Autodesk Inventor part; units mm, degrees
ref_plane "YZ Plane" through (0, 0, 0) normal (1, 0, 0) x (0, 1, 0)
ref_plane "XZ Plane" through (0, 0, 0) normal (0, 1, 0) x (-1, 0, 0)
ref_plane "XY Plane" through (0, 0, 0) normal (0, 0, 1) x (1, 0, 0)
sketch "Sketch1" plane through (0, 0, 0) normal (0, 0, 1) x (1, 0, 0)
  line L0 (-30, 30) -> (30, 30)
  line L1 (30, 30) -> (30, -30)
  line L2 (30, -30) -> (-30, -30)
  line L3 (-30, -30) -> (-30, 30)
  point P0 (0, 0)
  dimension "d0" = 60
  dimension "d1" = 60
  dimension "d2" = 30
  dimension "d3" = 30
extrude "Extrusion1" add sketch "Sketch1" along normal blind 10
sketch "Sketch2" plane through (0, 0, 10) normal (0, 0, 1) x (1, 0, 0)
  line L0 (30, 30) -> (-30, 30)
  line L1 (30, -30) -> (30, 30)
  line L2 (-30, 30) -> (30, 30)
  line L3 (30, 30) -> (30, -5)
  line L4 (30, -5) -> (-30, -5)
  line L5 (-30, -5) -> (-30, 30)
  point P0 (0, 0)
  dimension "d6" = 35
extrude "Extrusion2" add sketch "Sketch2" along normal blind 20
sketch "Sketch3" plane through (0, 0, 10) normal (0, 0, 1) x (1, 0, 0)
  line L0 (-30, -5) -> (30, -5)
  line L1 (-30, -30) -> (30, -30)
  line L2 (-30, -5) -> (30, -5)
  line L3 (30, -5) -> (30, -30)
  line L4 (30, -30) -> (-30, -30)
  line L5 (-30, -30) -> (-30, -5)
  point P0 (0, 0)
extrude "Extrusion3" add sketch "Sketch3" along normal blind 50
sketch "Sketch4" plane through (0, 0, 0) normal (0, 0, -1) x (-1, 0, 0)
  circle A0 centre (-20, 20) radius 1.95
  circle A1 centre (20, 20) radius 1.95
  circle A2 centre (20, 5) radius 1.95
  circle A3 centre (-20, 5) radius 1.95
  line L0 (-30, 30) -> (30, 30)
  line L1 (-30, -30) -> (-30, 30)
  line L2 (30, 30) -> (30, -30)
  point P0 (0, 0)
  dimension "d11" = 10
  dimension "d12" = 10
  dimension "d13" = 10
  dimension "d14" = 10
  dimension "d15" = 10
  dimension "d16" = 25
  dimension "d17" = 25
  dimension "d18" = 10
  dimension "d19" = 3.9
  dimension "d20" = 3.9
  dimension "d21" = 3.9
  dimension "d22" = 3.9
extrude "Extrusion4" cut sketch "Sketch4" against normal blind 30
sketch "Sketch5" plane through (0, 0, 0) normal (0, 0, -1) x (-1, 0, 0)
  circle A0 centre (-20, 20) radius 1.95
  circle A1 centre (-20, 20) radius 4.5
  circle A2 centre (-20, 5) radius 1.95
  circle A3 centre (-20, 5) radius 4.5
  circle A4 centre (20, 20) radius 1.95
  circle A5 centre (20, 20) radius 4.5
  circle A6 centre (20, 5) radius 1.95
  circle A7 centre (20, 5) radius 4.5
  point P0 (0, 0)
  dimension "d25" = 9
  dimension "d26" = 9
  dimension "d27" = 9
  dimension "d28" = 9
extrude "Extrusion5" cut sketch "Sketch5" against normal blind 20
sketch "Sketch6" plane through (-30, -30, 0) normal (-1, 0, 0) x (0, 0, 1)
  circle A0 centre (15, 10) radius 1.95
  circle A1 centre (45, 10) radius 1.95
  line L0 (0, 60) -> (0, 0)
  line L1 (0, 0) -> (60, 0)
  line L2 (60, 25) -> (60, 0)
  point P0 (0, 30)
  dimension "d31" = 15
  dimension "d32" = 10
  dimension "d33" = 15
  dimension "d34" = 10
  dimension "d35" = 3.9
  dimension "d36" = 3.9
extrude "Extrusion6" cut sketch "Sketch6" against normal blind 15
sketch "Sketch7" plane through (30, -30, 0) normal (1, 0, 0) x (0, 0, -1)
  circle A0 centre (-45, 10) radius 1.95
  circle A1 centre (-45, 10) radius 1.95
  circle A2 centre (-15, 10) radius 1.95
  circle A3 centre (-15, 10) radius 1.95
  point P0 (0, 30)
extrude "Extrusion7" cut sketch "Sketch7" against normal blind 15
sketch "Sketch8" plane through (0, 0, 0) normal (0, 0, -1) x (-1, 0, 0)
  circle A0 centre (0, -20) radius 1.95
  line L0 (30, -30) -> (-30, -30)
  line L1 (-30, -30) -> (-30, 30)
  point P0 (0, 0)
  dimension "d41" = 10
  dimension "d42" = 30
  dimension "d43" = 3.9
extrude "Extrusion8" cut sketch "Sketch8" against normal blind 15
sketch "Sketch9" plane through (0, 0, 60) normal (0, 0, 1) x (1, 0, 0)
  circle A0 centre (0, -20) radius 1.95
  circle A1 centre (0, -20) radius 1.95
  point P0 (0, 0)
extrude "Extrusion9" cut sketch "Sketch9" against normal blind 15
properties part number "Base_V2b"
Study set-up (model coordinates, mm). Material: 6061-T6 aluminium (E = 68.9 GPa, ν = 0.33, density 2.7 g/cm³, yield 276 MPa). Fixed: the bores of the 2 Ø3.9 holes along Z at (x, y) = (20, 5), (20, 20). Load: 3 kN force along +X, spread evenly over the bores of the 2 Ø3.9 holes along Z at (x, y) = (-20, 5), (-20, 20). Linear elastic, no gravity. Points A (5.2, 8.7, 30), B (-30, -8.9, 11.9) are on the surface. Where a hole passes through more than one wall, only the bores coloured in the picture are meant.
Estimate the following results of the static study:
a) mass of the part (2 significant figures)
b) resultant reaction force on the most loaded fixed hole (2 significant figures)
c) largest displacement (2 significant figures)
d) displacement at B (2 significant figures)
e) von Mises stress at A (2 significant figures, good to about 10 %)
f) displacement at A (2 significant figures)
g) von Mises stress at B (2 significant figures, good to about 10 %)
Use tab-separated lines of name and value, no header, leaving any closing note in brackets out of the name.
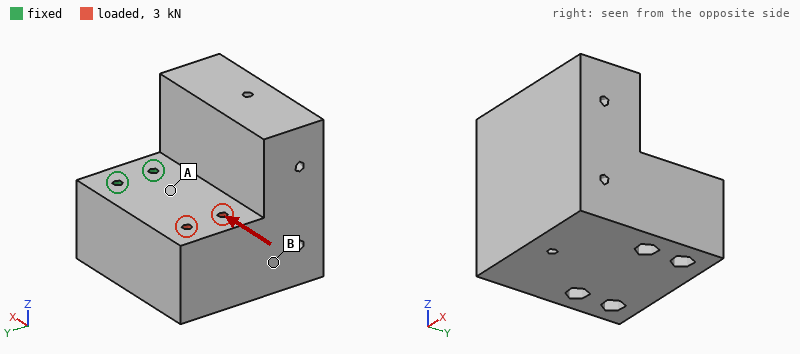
mass of the part	400 g
resultant reaction force on the most loaded fixed hole	1.5 kN
largest displacement	7.0 µm
displacement at B	3.8 µm
von Mises stress at A	7.9 MPa
displacement at A	2.0 µm
von Mises stress at B	2.1 MPa
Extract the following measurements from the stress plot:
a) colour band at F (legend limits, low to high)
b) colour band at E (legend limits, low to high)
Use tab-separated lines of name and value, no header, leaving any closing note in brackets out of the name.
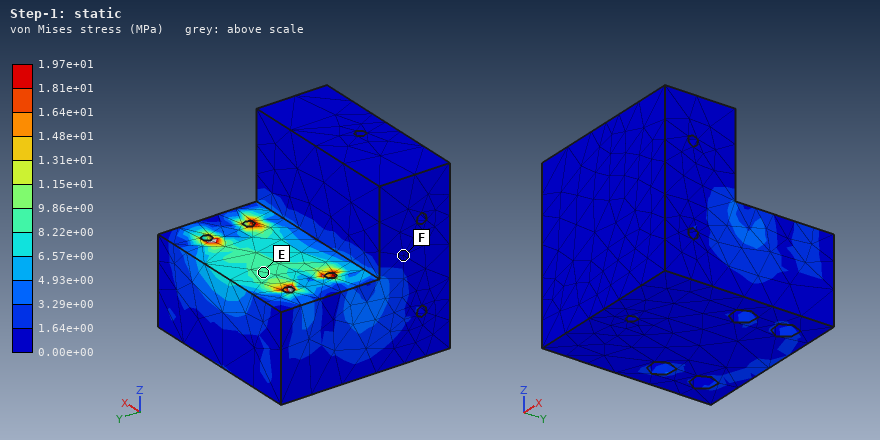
colour band at F	0.00e+00 to 1.64e+00 MPa
colour band at E	8.22e+00 to 9.86e+00 MPa
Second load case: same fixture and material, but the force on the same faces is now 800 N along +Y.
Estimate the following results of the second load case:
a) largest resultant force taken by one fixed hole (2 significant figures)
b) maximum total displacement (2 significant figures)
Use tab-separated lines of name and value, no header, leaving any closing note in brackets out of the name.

largest resultant force taken by one fixed hole	1.8 kN
maximum total displacement	18 µm
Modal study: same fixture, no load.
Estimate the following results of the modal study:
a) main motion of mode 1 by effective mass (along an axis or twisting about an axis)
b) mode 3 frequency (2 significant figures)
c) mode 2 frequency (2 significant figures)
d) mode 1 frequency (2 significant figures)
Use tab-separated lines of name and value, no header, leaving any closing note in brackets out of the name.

main motion of mode 1 by effective mass	along Z
mode 3 frequency	3100 Hz
mode 2 frequency	2400 Hz
mode 1 frequency	1600 Hz
